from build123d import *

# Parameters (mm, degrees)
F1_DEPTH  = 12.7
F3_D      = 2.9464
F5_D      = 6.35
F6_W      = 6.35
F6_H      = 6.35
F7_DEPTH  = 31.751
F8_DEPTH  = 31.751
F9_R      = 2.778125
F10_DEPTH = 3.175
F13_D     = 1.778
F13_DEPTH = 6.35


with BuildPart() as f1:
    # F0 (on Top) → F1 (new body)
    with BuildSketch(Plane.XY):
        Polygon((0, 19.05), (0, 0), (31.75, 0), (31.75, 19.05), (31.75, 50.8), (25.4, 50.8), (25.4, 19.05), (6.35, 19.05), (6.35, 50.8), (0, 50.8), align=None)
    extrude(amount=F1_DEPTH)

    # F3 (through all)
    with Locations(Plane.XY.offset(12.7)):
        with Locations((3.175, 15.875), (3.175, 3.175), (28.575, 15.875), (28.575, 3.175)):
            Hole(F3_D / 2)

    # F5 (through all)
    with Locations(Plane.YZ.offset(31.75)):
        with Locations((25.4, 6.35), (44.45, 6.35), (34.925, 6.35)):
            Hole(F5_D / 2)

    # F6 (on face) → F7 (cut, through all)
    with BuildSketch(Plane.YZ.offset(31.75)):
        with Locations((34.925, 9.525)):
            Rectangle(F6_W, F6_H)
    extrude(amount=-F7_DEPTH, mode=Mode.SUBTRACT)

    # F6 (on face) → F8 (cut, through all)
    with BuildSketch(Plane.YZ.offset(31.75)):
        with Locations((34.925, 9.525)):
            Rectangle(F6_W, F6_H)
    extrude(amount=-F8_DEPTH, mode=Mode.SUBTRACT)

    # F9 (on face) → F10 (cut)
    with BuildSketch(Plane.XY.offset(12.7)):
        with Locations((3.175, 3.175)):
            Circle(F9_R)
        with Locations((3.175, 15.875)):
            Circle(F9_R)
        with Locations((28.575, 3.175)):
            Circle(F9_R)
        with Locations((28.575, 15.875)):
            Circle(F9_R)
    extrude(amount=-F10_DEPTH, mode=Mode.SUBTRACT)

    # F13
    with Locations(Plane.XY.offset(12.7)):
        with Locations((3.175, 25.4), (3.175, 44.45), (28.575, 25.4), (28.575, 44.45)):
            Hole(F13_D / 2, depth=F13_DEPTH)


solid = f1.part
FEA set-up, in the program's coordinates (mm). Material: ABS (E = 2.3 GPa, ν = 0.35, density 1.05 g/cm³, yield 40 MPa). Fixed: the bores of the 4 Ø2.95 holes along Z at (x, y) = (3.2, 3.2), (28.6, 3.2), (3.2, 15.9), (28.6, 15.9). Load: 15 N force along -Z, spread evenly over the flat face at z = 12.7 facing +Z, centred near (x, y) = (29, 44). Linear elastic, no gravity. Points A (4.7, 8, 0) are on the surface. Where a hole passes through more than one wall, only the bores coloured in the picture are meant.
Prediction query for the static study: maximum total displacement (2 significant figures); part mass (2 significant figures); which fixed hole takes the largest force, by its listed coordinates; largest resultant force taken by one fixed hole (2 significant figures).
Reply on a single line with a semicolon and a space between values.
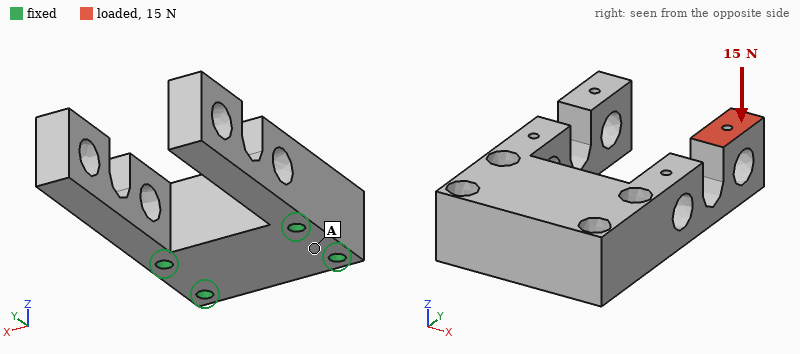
0.59 mm; 11 g; (28.6, 15.9); 23 N
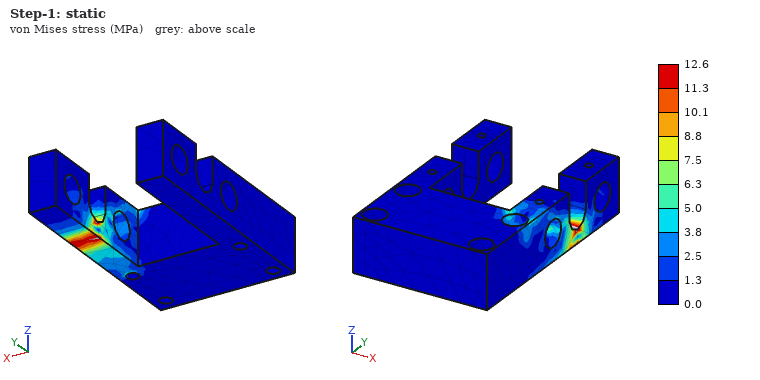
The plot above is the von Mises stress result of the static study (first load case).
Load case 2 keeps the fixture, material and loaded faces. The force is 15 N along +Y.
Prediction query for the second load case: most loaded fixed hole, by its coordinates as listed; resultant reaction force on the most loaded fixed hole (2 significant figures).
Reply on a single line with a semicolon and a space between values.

(28.6, 15.9); 12 N
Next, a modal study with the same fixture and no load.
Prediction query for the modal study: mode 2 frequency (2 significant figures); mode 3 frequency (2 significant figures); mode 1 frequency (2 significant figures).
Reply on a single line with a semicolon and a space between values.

980 Hz; 990 Hz; 980 Hz
